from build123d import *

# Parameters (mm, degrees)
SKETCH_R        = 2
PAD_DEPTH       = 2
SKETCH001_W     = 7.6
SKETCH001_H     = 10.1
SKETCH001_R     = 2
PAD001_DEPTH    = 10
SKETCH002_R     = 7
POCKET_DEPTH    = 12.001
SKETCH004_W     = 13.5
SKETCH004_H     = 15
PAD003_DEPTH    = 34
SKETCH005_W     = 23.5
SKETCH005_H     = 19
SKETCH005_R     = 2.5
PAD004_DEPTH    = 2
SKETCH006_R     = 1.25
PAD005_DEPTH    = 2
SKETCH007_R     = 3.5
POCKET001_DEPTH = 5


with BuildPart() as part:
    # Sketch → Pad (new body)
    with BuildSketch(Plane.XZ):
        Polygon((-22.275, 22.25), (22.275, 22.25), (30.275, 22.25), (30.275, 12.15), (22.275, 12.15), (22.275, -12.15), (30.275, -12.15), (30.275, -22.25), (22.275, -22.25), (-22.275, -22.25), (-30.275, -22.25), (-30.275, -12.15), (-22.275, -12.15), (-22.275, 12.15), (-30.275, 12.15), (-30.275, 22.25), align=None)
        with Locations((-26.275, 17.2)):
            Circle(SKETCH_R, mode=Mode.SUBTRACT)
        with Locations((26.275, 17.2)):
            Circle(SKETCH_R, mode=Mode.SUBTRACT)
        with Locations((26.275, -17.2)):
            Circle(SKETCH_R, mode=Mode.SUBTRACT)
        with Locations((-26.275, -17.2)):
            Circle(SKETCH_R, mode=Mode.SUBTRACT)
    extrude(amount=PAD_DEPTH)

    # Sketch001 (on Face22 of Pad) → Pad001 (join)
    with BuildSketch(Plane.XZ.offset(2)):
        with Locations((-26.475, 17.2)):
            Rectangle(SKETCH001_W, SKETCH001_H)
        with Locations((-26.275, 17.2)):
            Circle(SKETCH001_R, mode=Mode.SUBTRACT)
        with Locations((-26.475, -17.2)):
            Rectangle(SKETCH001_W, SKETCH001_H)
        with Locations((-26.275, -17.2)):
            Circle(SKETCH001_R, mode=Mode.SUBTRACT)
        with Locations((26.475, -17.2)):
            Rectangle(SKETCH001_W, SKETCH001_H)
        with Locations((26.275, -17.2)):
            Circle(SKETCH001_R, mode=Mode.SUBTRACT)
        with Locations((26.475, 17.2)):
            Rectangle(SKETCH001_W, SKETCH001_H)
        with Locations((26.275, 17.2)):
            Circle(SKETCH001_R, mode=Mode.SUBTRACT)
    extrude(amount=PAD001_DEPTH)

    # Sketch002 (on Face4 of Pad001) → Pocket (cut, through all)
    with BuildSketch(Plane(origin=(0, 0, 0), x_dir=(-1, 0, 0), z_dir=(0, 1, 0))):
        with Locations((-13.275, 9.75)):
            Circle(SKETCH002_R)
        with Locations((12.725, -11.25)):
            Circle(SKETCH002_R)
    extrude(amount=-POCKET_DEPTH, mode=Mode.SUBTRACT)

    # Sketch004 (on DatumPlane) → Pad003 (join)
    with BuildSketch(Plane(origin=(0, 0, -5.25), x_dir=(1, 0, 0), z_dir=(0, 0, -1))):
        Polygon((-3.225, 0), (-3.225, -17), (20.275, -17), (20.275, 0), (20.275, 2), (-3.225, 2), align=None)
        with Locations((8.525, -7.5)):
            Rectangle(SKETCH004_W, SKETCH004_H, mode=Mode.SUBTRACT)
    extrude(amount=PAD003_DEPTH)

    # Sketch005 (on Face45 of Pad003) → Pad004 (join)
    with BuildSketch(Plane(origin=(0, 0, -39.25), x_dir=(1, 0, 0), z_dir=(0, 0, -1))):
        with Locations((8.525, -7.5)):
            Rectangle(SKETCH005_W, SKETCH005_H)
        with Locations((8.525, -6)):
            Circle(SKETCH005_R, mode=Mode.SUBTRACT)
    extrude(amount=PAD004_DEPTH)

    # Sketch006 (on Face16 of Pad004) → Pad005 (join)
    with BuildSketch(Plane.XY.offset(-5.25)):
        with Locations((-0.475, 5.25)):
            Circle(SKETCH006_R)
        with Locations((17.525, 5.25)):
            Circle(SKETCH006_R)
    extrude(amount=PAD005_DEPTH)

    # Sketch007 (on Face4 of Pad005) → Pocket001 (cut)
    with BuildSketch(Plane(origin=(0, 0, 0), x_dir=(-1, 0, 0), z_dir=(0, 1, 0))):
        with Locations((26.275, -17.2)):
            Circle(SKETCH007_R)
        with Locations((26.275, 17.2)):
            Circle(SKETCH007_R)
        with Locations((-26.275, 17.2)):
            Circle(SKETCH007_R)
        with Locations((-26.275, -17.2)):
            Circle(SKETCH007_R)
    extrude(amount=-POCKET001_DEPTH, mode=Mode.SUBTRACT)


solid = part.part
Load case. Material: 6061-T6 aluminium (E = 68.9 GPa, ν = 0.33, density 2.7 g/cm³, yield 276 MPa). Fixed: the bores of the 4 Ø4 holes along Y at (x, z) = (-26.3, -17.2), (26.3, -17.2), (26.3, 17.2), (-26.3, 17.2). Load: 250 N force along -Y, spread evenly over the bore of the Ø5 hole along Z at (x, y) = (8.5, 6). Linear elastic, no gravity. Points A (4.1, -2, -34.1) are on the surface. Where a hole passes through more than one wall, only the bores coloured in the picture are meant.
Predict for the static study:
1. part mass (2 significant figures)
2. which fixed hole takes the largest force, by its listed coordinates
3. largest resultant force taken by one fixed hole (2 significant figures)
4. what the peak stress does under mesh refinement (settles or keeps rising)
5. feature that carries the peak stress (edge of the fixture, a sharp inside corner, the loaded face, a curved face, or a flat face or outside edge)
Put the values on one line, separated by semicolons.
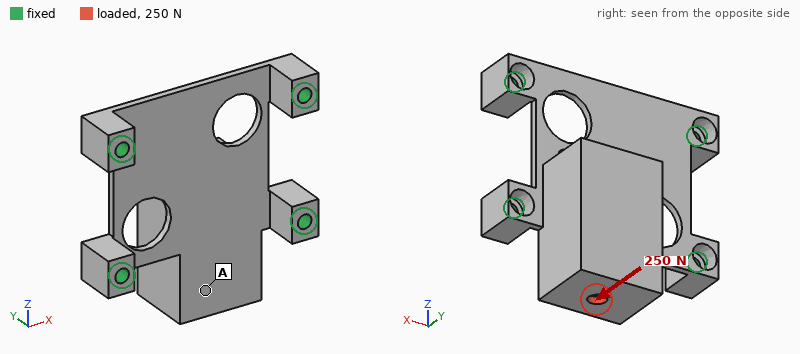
39 g; (26.3, -17.2); 260 N; keeps rising; a sharp inside corner
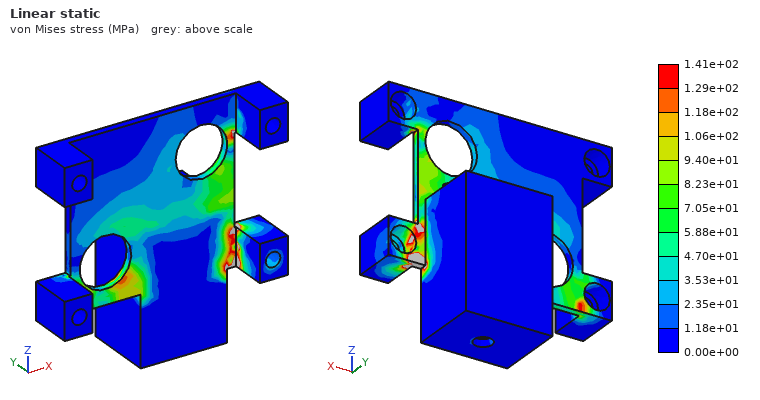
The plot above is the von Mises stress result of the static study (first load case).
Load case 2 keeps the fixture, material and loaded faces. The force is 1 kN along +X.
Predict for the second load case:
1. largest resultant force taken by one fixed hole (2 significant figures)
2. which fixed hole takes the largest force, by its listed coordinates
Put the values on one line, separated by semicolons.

740 N; (26.3, -17.2)
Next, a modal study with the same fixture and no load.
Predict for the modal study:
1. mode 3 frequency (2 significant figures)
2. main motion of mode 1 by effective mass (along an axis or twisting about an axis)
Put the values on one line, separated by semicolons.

5100 Hz; along Y
